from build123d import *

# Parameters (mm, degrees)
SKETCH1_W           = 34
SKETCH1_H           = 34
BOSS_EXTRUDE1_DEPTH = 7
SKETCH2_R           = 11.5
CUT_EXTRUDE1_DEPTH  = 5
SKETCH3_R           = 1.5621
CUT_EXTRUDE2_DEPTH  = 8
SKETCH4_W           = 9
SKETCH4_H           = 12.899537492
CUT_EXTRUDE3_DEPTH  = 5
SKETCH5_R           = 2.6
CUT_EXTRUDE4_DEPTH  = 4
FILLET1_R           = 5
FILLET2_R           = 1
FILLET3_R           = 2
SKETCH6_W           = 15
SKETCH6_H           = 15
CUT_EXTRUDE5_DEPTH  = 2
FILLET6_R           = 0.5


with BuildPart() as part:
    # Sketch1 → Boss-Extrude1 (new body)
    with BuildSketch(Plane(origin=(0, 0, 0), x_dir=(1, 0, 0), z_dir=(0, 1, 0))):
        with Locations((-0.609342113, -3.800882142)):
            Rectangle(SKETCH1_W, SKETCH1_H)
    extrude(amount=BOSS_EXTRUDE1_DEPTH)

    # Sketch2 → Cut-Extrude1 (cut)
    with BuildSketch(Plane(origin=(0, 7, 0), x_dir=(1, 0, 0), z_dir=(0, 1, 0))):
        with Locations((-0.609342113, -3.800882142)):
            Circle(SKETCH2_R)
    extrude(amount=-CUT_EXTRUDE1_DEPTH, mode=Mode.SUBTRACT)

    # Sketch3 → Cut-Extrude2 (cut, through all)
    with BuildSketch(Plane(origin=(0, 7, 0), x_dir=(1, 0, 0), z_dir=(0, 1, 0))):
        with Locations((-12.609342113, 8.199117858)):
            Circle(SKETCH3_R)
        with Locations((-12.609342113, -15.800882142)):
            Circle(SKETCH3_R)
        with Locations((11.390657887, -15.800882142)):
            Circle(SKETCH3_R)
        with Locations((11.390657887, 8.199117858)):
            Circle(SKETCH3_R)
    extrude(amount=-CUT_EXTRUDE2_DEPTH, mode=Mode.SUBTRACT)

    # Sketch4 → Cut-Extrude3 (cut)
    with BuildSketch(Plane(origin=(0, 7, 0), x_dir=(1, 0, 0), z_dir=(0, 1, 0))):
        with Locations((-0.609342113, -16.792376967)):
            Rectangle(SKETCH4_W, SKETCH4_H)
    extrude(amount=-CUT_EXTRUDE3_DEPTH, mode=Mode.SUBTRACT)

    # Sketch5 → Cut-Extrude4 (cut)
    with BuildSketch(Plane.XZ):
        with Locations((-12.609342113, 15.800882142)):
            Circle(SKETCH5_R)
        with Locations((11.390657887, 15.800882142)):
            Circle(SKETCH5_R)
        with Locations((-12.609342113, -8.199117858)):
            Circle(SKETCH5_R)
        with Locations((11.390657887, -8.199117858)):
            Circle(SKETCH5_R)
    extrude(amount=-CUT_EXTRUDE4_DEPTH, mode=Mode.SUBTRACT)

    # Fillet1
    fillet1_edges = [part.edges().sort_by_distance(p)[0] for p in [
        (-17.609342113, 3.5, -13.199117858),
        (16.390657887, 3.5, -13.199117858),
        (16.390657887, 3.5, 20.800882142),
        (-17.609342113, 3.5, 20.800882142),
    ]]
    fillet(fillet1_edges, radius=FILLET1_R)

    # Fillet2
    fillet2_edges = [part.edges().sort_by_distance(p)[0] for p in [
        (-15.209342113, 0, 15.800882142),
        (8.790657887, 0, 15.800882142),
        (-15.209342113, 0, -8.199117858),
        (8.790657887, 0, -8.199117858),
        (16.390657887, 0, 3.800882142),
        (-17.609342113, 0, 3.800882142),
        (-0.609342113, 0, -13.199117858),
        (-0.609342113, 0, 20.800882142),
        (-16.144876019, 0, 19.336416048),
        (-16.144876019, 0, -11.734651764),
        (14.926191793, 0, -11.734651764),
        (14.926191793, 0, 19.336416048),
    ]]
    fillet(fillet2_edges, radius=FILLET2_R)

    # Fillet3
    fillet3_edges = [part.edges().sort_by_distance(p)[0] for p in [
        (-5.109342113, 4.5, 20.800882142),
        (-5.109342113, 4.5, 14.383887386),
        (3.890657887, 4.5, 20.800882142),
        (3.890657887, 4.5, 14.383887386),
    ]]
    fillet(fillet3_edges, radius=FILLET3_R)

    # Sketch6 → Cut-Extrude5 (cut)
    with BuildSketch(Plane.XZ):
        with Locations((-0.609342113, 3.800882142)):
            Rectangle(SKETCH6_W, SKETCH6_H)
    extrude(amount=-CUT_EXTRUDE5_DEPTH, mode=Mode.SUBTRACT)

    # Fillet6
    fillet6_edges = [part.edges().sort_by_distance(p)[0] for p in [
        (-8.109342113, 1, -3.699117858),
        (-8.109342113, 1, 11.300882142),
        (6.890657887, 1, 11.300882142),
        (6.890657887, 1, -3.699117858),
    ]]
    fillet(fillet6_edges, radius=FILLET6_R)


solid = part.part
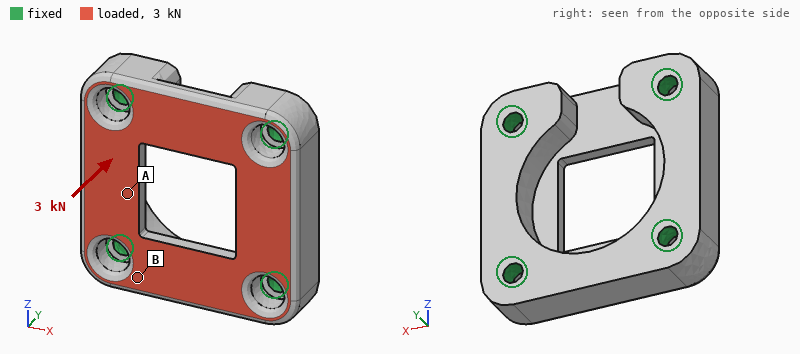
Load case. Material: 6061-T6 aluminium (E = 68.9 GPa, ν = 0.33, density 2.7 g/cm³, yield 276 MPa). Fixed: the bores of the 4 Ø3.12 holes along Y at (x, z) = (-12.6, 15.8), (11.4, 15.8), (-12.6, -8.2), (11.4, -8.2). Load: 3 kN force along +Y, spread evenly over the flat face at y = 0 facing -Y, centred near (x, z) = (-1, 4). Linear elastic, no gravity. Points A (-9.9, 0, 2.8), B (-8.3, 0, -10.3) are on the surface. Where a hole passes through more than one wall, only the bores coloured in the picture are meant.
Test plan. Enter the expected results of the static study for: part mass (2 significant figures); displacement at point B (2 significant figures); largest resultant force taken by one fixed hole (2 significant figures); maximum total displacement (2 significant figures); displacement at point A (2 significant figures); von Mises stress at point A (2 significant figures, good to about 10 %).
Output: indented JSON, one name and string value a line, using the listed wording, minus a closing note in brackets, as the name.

{
  "part mass": "13 g",
  "displacement at point B": "3.9 µm",
  "largest resultant force taken by one fixed hole": "870 N",
  "maximum total displacement": "19 µm",
  "displacement at point A": "11 µm",
  "von Mises stress at point A": "34 MPa"
}
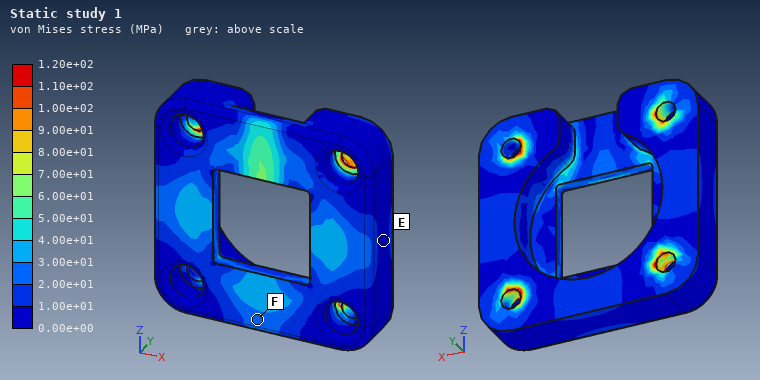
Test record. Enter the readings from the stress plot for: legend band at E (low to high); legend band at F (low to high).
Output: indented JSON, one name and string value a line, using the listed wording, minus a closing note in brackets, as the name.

{
  "legend band at E": "0.00e+00 to 1.00e+01 MPa",
  "legend band at F": "2.00e+01 to 3.00e+01 MPa"
}
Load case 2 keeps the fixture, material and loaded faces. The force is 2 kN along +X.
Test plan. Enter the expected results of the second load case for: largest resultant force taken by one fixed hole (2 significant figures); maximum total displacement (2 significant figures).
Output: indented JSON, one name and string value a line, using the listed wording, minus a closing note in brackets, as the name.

{
  "largest resultant force taken by one fixed hole": "560 N",
  "maximum total displacement": "11 µm"
}
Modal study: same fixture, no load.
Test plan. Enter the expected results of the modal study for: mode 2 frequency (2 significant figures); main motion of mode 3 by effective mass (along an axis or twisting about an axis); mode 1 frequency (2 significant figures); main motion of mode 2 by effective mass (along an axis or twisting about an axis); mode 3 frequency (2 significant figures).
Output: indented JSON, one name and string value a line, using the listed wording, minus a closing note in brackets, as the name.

{
  "mode 2 frequency": "34 kHz",
  "main motion of mode 3 by effective mass": "along Y",
  "mode 1 frequency": "31 kHz",
  "main motion of mode 2 by effective mass": "along X",
  "mode 3 frequency": "37 kHz"
}
